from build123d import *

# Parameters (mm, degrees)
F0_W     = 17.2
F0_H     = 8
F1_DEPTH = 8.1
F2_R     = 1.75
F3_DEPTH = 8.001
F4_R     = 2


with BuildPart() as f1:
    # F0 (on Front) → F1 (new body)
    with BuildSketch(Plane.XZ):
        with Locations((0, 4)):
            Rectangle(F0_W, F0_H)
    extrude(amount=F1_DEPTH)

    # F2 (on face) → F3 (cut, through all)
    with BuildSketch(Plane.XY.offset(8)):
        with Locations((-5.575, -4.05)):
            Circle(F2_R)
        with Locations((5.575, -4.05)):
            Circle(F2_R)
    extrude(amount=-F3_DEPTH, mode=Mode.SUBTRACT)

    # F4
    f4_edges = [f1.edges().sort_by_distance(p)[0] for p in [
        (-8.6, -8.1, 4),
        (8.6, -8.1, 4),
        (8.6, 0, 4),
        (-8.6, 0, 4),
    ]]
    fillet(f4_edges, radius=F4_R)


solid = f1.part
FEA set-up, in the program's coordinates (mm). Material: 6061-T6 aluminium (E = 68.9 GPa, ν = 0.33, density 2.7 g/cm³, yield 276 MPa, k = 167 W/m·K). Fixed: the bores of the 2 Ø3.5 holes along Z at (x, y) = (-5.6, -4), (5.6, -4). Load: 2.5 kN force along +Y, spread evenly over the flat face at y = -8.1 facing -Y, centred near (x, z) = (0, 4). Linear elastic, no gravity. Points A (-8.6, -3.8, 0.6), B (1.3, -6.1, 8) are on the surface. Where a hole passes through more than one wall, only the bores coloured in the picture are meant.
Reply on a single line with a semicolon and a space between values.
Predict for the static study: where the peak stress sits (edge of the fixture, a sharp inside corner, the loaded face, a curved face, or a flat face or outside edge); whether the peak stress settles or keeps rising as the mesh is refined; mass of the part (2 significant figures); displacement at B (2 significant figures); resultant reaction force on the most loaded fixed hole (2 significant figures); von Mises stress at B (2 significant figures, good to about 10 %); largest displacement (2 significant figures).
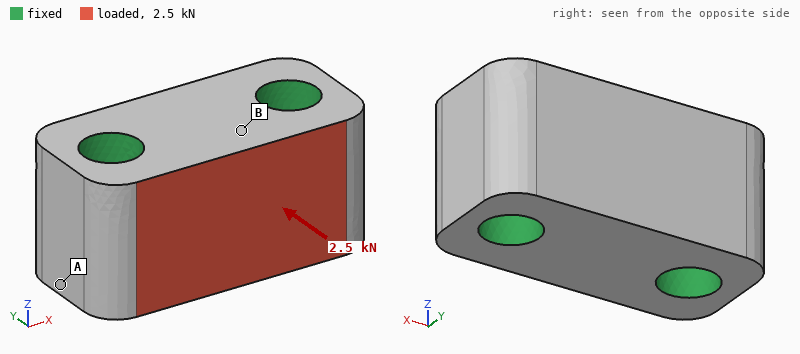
edge of the fixture; keeps rising; 2.5 g; 2.0 µm; 1.3 kN; 18 MPa; 2.7 µm
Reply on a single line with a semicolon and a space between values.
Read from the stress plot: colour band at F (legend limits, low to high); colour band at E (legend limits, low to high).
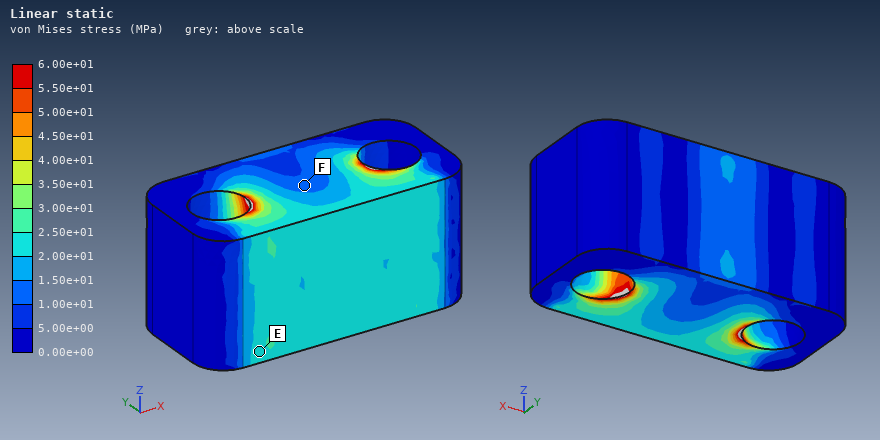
1.00e+01 to 1.50e+01 MPa; 2.00e+01 to 2.50e+01 MPa
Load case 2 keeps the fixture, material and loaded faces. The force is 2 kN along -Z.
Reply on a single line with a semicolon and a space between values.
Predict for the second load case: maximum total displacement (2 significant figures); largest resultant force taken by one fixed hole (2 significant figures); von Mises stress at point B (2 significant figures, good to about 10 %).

6.6 µm; 1.0 kN; 29 MPa
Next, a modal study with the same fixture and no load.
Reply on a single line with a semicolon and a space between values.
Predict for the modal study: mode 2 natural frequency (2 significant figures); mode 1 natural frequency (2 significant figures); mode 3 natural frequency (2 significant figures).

150 kHz; 140 kHz; 150 kHz
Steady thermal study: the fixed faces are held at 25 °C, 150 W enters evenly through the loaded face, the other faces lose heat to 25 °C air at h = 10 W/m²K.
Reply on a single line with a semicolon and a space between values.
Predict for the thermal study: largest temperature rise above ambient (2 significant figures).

35 K
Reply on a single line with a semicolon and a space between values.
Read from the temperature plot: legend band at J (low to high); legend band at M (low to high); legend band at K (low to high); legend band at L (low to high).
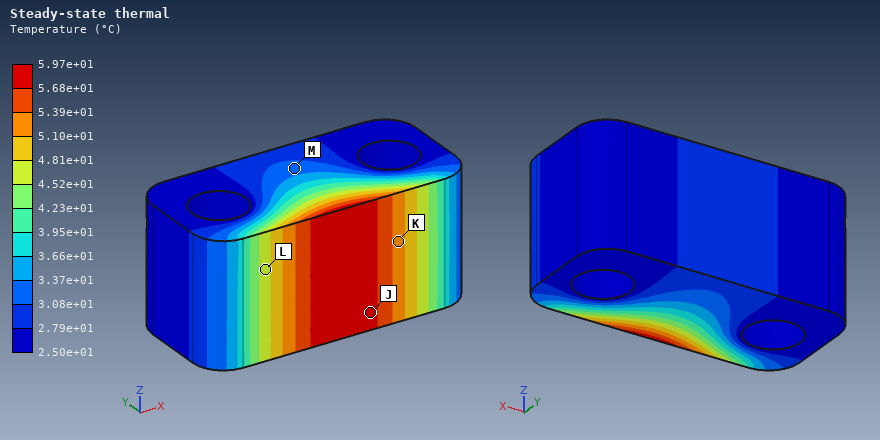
5.68e+01 to 5.97e+01 °C; 3.08e+01 to 3.37e+01 °C; 5.10e+01 to 5.39e+01 °C; 4.52e+01 to 4.81e+01 °C
